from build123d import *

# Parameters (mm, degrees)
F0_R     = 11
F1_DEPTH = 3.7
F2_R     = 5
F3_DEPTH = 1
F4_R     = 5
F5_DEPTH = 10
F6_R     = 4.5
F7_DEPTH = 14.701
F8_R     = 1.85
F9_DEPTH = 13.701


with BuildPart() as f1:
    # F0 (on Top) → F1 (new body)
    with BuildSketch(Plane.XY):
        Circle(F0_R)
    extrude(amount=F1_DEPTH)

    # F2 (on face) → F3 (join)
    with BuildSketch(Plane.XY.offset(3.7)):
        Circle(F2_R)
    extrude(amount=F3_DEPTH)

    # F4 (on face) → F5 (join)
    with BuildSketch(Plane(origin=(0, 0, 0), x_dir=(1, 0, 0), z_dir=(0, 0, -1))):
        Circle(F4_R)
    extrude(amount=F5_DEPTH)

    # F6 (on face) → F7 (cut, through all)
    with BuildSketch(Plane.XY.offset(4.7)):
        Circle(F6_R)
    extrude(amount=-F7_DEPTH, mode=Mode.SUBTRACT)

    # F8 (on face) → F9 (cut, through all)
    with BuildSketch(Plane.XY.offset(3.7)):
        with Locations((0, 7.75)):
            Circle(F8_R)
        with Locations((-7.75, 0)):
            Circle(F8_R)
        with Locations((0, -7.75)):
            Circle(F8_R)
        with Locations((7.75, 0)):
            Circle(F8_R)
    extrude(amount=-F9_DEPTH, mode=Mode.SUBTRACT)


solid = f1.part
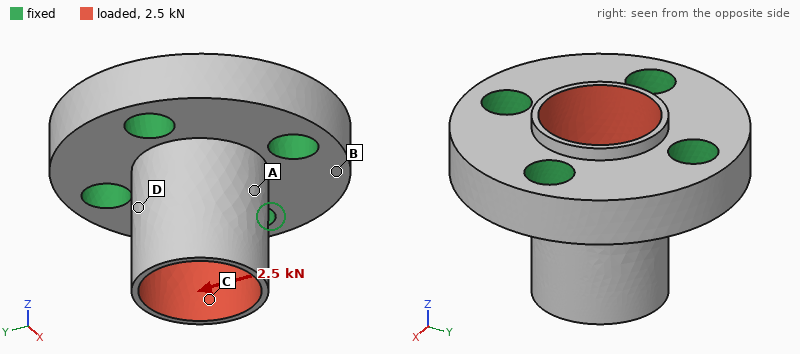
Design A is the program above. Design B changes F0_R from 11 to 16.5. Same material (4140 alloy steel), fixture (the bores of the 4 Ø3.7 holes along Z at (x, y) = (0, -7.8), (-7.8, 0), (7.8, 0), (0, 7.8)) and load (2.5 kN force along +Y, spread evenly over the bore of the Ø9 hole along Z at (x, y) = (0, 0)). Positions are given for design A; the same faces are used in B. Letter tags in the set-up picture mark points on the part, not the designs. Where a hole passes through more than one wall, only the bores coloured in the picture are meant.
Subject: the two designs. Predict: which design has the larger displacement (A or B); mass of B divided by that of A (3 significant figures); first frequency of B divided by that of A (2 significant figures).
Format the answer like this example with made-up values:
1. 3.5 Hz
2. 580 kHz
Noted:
1. A
2. 2.49
3. 0.62
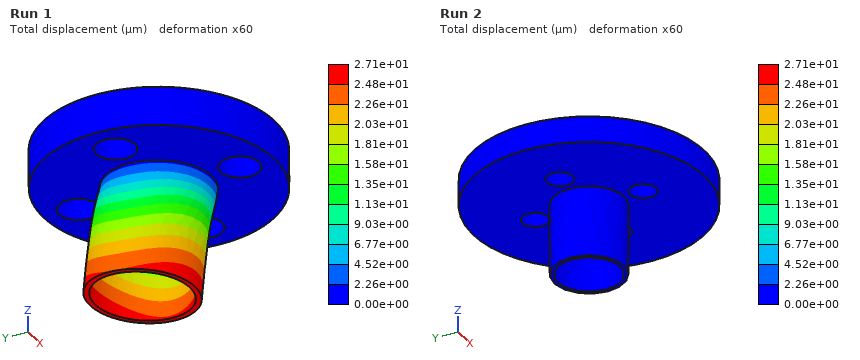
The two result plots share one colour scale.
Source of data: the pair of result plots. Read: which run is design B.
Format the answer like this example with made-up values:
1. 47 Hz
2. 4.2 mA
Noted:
1. Run 2
